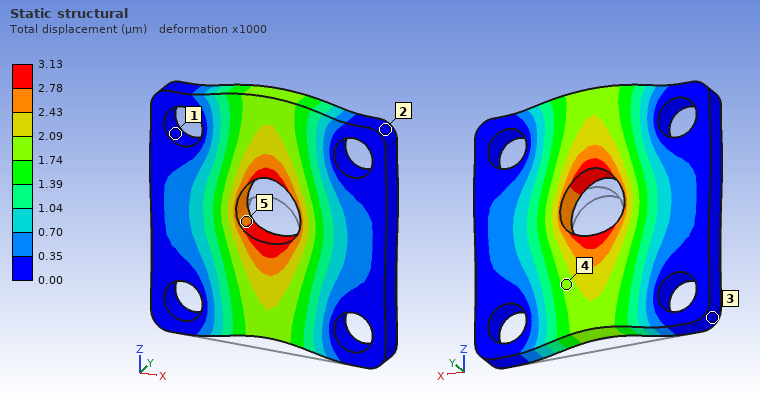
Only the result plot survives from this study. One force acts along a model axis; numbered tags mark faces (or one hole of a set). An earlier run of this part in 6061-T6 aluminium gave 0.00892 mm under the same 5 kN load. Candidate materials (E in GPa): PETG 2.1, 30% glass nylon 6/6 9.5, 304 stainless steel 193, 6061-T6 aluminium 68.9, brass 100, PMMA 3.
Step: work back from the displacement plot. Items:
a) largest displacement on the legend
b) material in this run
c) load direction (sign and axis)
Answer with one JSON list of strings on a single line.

["3.13 µm", "304 stainless steel", "+Z"]
